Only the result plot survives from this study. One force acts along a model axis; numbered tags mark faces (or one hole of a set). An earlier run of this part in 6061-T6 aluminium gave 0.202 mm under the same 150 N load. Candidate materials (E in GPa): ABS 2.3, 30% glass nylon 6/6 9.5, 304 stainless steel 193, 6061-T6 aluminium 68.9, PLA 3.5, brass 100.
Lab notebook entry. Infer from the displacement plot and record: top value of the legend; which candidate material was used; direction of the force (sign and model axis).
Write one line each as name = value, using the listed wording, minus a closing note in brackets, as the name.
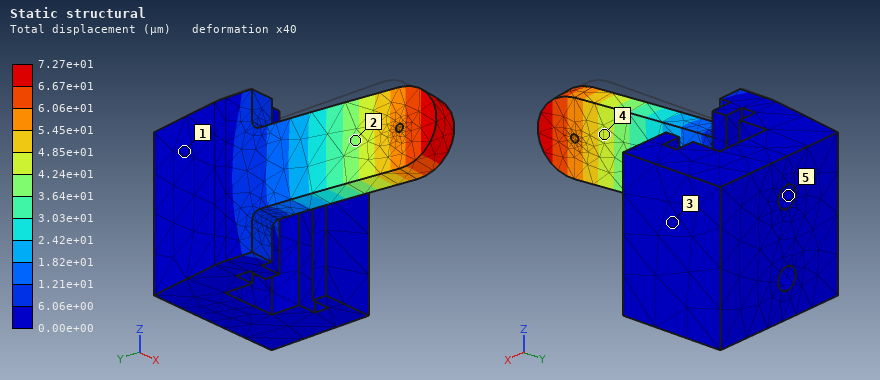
top value of the legend = 7.27e+01 µm
which candidate material was used = 304 stainless steel
direction of the force = +X
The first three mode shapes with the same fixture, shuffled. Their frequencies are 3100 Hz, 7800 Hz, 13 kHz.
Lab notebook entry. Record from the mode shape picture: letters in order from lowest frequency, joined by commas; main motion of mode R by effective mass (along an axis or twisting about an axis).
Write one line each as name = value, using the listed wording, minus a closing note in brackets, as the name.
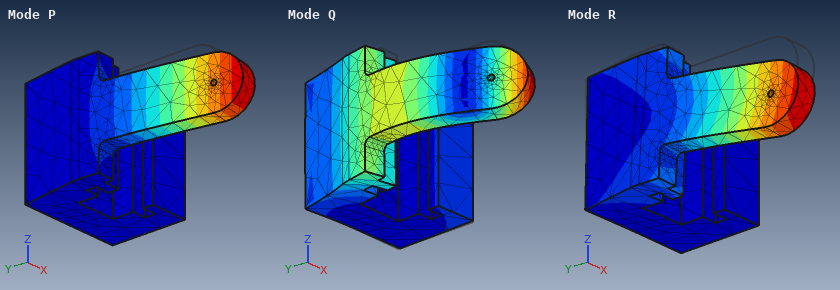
letters in order from lowest frequency, joined by commas = P, R, Q
main motion of mode R by effective mass = along Z
